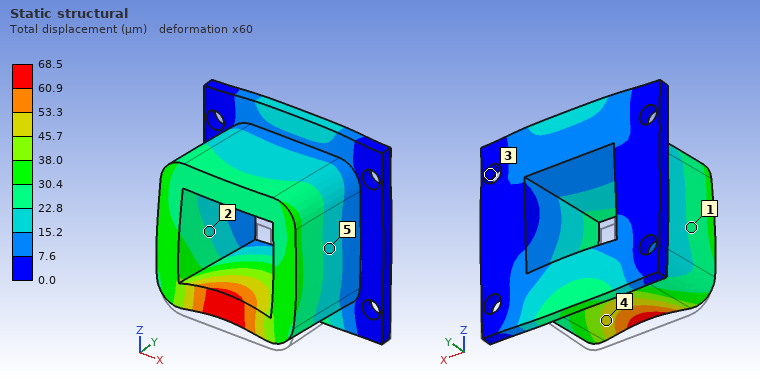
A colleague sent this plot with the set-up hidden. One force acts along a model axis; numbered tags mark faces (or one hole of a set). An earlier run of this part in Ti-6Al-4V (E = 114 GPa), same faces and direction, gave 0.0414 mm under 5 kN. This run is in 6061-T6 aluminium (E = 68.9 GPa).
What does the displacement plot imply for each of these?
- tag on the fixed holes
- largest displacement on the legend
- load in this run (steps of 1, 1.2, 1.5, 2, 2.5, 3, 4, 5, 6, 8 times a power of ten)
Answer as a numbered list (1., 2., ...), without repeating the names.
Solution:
1. 3
2. 68.5 µm
3. 5 kN
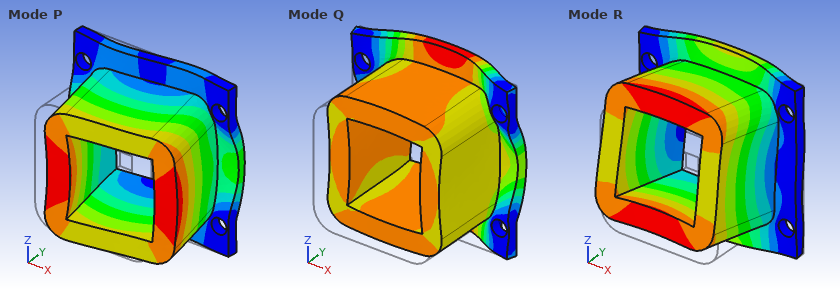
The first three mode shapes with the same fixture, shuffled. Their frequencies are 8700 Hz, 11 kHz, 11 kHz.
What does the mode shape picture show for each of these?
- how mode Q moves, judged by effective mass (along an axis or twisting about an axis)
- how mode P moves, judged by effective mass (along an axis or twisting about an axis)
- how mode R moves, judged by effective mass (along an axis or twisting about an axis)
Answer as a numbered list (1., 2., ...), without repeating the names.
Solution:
1. along Y
2. along X
3. along Z
